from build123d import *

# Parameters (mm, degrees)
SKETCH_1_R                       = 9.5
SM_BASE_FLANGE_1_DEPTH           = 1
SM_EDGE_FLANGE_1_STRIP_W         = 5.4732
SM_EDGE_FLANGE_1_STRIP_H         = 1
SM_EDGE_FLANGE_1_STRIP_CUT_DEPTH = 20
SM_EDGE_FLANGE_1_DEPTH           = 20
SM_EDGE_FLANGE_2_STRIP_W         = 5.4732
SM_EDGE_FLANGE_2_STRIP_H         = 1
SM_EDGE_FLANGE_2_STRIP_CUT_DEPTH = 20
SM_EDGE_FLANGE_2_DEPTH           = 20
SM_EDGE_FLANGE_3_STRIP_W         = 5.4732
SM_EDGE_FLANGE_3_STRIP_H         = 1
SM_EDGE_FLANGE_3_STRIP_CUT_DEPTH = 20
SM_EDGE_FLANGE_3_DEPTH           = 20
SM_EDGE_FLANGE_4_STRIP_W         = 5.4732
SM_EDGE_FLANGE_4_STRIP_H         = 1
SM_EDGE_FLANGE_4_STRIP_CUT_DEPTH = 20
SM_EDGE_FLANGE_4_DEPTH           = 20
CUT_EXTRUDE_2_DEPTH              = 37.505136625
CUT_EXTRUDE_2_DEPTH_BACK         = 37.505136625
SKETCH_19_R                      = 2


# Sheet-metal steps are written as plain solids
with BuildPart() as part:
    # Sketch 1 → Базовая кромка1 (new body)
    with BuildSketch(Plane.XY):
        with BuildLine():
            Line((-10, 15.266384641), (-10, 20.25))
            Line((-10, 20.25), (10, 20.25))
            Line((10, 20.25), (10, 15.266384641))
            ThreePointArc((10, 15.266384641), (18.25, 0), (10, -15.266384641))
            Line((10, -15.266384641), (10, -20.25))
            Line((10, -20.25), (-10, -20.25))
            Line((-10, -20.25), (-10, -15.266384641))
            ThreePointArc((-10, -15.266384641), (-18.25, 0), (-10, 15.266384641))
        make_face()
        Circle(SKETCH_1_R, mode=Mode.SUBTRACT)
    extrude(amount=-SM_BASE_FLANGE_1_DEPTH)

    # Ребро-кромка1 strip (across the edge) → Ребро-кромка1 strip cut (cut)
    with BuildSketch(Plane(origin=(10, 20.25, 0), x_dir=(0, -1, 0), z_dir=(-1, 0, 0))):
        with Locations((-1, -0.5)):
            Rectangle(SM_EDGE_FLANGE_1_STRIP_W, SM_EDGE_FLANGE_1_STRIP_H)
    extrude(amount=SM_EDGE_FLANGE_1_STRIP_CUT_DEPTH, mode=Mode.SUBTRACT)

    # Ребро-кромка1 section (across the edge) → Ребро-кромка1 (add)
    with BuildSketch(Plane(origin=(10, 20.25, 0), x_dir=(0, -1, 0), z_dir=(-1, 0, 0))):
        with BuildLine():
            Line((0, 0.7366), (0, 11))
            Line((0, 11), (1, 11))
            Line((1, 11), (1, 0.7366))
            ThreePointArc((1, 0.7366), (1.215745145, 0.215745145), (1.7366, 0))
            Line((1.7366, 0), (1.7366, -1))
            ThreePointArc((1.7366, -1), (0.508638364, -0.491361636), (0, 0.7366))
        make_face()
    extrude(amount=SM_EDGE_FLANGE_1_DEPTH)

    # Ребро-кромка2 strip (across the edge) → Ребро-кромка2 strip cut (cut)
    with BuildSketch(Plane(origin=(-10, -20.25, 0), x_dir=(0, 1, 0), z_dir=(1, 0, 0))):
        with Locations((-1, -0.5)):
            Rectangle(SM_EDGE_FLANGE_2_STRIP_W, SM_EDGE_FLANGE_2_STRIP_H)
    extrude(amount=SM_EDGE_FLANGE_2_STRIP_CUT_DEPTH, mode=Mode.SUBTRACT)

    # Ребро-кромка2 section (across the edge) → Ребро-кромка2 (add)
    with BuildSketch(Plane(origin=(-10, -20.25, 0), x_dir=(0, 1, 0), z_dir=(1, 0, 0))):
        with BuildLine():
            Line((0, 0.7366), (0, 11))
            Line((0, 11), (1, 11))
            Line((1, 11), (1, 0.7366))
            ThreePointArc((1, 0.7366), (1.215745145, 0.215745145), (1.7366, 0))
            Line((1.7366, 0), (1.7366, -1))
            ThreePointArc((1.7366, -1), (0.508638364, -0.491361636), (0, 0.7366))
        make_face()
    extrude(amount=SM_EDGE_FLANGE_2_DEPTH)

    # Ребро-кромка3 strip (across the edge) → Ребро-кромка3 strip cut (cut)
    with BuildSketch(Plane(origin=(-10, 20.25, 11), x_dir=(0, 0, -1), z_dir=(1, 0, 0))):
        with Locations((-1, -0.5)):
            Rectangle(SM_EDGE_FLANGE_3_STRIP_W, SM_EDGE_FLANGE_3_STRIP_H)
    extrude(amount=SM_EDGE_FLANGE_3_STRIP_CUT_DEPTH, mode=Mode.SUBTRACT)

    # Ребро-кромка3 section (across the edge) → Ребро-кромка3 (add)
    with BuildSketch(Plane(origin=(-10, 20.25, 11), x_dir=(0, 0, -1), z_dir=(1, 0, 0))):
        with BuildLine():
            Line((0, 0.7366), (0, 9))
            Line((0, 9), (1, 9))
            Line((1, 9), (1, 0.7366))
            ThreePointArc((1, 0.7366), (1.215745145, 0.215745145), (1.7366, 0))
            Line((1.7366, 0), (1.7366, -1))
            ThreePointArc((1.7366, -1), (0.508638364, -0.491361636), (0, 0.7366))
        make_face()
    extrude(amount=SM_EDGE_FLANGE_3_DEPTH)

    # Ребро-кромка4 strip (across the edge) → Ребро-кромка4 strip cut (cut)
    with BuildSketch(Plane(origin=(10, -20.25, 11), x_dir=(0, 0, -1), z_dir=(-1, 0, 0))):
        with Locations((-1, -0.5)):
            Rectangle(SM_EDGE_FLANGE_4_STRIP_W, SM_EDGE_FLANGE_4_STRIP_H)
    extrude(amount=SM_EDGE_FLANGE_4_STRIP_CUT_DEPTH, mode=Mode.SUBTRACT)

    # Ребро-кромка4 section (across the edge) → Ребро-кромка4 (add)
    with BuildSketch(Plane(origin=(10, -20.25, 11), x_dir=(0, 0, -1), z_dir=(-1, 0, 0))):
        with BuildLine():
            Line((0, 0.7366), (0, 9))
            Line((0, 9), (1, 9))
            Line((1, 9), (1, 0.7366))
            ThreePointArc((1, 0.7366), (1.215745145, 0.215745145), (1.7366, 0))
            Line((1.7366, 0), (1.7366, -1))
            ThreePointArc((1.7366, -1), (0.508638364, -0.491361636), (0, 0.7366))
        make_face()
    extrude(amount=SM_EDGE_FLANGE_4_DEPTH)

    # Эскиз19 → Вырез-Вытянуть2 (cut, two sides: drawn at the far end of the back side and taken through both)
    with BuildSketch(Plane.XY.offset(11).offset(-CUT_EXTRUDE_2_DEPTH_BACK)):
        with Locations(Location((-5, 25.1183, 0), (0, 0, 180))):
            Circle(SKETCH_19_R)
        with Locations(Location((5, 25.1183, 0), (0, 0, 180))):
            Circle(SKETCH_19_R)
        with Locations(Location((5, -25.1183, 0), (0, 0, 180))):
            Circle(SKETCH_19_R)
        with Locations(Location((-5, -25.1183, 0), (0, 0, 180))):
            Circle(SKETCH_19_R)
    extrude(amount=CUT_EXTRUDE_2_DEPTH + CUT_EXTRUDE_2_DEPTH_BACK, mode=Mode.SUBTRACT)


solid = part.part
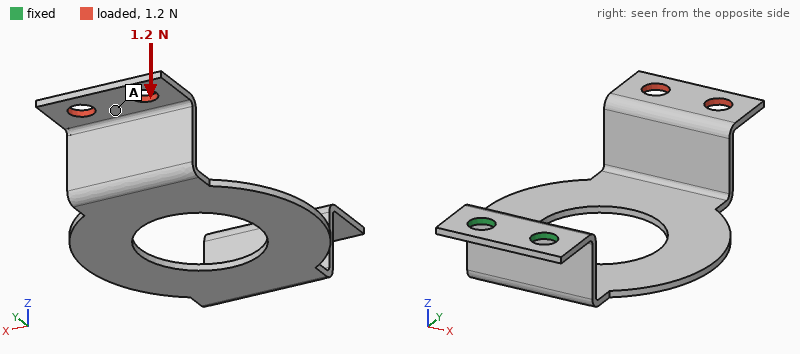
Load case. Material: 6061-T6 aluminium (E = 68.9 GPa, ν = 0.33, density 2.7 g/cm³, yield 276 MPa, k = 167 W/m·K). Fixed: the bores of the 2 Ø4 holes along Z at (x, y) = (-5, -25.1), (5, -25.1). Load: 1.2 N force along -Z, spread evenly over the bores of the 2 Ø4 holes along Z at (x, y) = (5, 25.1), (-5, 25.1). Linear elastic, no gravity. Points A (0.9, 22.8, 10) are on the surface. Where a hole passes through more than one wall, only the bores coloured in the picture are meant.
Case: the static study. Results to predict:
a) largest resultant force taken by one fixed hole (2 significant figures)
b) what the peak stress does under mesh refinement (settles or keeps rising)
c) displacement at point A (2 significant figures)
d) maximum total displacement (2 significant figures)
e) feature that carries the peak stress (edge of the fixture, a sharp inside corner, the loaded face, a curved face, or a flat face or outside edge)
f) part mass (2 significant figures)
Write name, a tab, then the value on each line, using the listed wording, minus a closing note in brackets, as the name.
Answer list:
largest resultant force taken by one fixed hole	0.70 N
what the peak stress does under mesh refinement	keeps rising
displacement at point A	0.59 mm
maximum total displacement	0.71 mm
feature that carries the peak stress	edge of the fixture
part mass	4.3 g
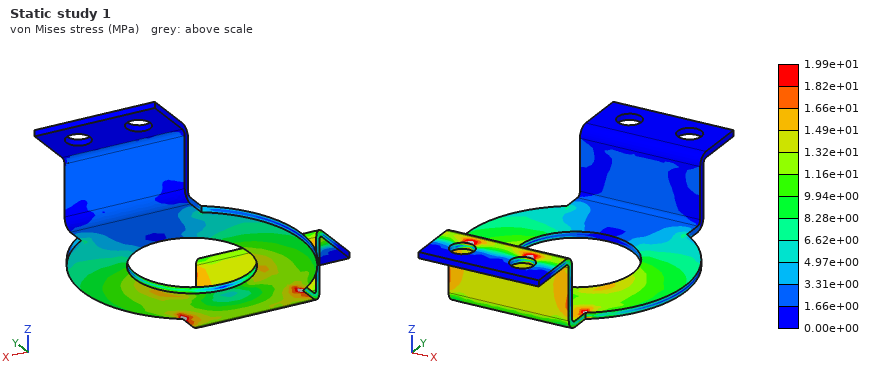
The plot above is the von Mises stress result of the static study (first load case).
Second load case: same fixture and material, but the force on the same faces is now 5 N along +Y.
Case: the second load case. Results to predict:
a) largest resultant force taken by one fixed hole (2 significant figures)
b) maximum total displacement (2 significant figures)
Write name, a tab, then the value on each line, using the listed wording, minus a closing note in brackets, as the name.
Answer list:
largest resultant force taken by one fixed hole	2.5 N
maximum total displacement	0.78 mm
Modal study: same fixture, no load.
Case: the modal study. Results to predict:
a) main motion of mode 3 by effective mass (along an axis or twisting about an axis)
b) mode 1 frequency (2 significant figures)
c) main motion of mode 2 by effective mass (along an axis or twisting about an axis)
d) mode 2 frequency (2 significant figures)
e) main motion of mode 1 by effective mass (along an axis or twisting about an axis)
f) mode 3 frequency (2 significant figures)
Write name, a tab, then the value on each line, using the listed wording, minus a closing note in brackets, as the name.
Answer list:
main motion of mode 3 by effective mass	along Y
mode 1 frequency	190 Hz
main motion of mode 2 by effective mass	along X
mode 2 frequency	430 Hz
main motion of mode 1 by effective mass	along Z
mode 3 frequency	890 Hz
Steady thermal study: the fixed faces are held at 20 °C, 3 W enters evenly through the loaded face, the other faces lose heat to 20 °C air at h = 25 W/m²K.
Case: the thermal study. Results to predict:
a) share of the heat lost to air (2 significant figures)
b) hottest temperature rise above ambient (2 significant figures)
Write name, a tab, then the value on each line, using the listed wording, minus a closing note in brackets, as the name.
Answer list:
share of the heat lost to air	54 %
hottest temperature rise above ambient	44 K
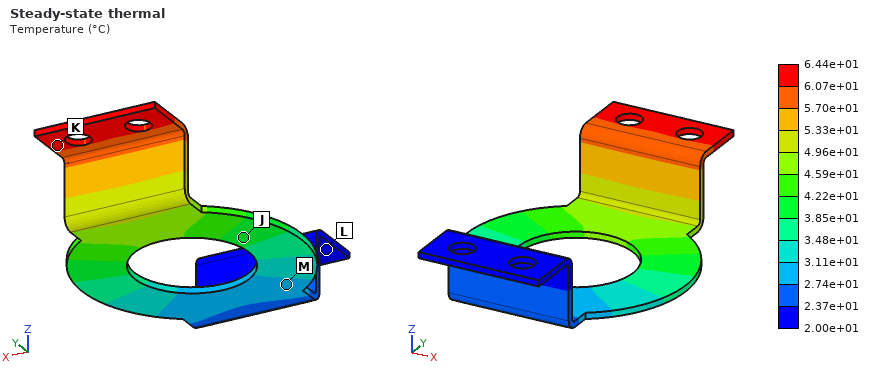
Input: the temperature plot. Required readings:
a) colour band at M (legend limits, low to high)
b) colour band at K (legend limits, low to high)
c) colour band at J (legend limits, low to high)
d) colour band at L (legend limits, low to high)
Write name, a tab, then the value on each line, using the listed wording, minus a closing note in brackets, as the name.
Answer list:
colour band at M	2.74e+01 to 3.11e+01 °C
colour band at K	6.07e+01 to 6.44e+01 °C
colour band at J	3.85e+01 to 4.22e+01 °C
colour band at L	2.00e+01 to 2.37e+01 °C
